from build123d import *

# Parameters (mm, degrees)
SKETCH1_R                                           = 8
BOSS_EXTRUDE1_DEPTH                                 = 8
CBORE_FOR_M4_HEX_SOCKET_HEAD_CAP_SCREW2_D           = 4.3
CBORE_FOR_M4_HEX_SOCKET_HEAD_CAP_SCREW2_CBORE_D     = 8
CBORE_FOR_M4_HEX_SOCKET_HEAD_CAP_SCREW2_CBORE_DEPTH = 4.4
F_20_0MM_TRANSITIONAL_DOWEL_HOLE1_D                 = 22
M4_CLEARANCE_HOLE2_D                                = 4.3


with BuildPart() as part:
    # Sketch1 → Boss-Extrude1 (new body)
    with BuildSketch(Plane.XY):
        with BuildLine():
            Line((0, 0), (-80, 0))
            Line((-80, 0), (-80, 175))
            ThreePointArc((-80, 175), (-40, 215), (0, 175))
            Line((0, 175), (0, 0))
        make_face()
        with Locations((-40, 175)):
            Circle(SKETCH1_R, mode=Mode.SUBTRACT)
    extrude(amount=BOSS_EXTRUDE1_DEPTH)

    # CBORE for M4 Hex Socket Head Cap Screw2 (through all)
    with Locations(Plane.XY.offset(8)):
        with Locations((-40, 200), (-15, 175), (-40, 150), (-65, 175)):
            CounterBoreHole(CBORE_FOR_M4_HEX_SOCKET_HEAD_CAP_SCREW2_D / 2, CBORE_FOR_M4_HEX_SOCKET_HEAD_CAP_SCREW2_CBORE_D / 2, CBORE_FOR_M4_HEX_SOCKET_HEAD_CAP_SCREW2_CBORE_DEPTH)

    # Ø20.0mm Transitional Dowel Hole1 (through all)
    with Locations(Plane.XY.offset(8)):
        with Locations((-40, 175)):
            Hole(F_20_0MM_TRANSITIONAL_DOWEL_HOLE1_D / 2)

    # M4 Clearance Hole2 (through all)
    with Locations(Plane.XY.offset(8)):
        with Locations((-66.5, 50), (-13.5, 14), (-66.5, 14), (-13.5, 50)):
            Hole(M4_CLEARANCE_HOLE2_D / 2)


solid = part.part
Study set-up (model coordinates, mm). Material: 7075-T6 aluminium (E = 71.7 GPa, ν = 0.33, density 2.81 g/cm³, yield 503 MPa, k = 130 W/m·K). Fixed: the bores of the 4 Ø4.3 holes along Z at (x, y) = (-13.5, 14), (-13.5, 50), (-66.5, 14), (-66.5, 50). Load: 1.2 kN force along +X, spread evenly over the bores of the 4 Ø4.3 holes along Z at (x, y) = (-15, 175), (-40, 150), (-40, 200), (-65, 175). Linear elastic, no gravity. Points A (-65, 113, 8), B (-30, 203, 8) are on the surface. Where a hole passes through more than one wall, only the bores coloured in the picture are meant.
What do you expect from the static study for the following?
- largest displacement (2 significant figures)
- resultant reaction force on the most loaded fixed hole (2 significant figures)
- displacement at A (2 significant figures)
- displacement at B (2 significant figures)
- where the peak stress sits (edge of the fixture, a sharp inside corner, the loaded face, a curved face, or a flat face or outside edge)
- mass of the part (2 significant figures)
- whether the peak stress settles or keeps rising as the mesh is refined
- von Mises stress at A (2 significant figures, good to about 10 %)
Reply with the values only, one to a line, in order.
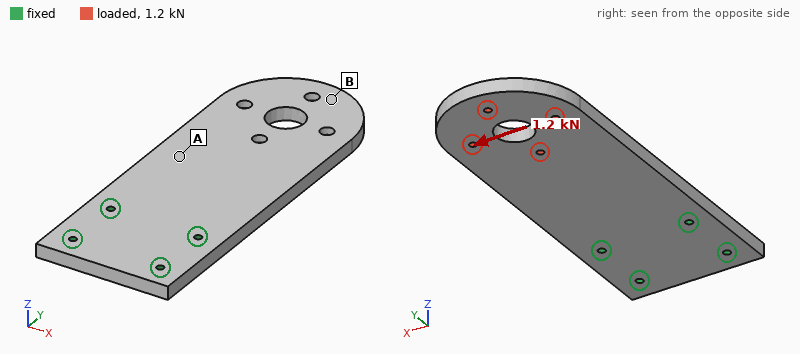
71 µm
2.3 kN
21 µm
60 µm
edge of the fixture
360 g
keeps rising
5.4 MPa
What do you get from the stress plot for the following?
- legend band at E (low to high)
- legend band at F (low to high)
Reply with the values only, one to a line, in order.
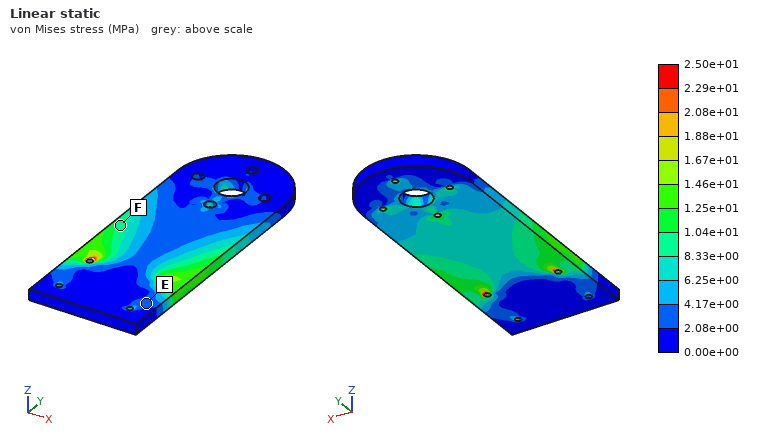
2.08e+00 to 4.17e+00 MPa
8.33e+00 to 1.04e+01 MPa
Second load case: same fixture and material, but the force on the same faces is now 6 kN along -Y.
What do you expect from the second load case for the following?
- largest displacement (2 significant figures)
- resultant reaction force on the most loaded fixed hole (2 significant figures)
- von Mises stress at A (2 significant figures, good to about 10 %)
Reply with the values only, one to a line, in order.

0.72 mm
2.3 kN
5.9 MPa
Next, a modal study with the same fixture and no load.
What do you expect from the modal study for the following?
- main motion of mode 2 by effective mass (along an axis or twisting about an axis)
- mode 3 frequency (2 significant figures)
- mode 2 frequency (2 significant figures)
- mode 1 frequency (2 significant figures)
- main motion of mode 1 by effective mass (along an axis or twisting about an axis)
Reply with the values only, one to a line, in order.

twisting about Y
1500 Hz
1100 Hz
270 Hz
along Z
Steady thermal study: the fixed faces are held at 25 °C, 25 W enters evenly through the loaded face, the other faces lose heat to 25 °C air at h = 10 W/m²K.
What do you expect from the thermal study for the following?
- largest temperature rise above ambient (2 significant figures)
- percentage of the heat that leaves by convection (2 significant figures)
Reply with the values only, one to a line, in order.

37 K
23 %
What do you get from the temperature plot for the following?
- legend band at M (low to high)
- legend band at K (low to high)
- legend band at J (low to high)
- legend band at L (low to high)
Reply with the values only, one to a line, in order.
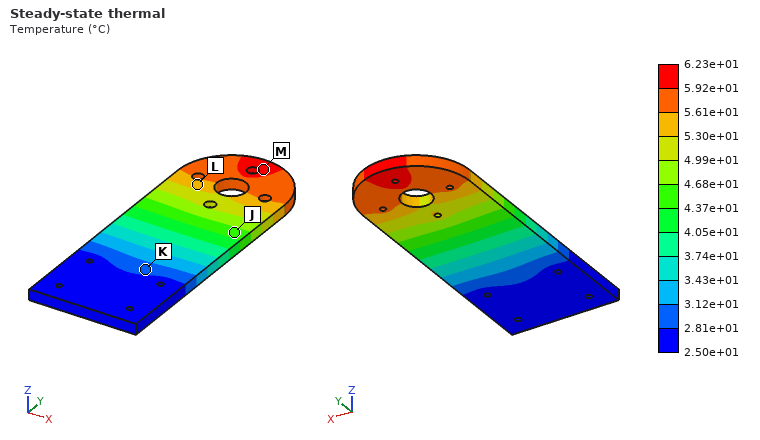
5.92e+01 to 6.23e+01 °C
2.81e+01 to 3.12e+01 °C
4.37e+01 to 4.68e+01 °C
5.30e+01 to 5.61e+01 °C
